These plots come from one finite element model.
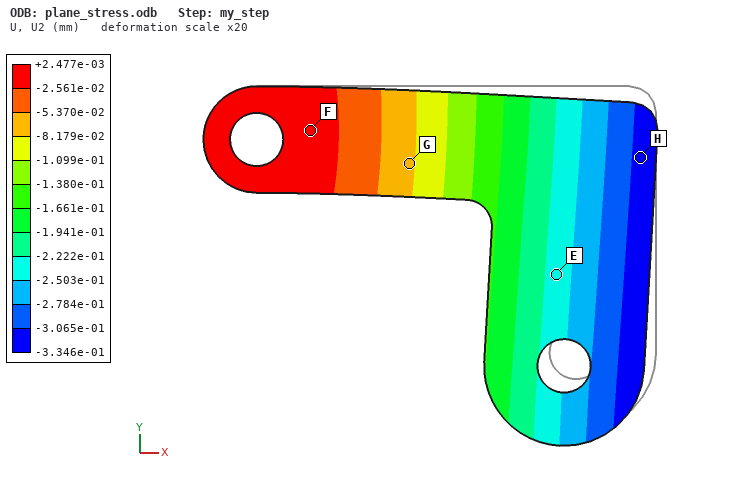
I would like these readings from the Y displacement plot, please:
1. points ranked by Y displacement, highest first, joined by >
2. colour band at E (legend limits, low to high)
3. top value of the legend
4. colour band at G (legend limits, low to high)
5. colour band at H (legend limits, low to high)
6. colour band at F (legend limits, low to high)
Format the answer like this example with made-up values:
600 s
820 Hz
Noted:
F > G > E > H
-2.503e-01 to -2.222e-01 mm
+2.477e-03 mm
-8.179e-02 to -5.370e-02 mm
-3.346e-01 to -3.065e-01 mm
-2.561e-02 to +2.477e-03 mm
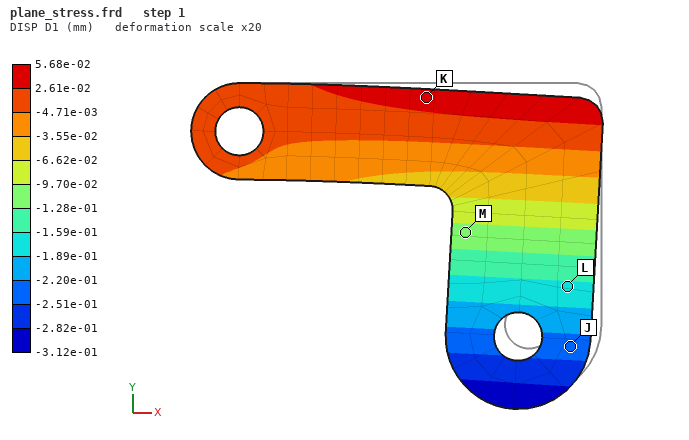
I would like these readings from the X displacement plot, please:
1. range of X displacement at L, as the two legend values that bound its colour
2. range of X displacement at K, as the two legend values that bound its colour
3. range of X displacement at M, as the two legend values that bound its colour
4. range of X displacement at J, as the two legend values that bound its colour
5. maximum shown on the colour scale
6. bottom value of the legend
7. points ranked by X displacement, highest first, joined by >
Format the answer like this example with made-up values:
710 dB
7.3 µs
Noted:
-1.89e-01 to -1.59e-01 mm
2.61e-02 to 5.68e-02 mm
-1.28e-01 to -9.70e-02 mm
-2.51e-01 to -2.20e-01 mm
5.68e-02 mm
-3.12e-01 mm
K > M > L > J
